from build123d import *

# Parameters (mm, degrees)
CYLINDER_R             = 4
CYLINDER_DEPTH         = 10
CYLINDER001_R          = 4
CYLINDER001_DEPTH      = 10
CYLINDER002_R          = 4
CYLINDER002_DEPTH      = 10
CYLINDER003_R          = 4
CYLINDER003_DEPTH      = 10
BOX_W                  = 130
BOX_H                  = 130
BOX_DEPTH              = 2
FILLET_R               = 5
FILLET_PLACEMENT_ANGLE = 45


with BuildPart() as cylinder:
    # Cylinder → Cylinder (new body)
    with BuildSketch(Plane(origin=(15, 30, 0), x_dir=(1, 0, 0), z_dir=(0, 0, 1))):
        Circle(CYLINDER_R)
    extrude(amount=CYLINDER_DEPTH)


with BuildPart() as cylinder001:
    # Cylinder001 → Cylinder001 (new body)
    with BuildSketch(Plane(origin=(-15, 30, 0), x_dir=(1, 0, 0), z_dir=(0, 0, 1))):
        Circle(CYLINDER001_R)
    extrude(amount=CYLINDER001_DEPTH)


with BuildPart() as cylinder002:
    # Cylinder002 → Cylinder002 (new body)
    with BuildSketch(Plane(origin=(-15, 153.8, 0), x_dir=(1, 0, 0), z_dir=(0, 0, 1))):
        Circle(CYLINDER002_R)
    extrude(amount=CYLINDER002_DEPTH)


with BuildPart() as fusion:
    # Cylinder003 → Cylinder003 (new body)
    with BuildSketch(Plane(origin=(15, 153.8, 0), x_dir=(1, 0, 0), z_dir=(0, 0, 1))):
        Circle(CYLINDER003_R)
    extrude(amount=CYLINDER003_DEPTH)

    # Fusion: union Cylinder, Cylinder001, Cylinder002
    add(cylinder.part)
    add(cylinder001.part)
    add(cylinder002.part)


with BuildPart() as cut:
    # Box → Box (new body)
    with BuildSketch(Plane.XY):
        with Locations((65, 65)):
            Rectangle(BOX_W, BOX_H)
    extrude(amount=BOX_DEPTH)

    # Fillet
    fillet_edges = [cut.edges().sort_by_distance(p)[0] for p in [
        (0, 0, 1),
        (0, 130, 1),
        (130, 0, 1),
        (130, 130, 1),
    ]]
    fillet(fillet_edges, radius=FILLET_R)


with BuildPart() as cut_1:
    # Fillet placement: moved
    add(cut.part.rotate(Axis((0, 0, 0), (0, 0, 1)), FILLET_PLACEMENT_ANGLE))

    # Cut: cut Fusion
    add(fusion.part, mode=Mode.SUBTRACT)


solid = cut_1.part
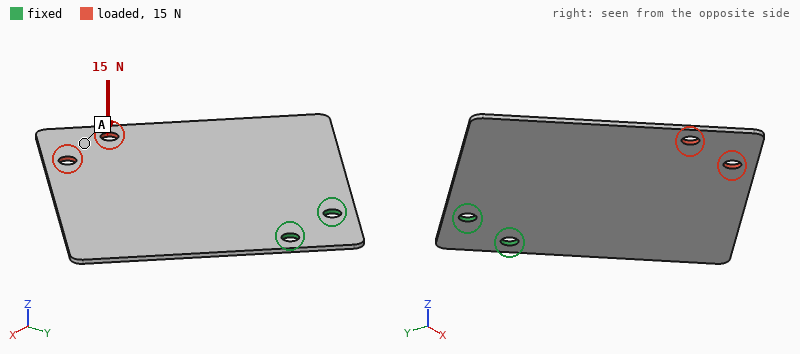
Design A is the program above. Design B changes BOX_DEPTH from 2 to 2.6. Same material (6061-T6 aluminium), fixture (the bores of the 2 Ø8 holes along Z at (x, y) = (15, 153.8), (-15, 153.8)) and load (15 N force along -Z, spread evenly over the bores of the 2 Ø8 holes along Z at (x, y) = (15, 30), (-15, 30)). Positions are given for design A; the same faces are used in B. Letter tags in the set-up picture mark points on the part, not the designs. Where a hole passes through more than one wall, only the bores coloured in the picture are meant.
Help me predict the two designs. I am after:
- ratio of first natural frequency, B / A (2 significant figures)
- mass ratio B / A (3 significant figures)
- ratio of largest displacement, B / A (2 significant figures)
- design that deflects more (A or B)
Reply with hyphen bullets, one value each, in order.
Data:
- 1.3
- 1.30
- 0.46
- A
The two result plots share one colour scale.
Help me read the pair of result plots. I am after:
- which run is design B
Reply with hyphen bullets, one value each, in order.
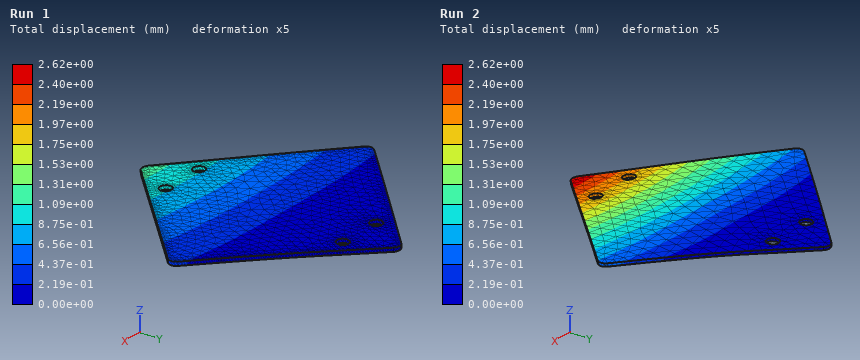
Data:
- Run 1
